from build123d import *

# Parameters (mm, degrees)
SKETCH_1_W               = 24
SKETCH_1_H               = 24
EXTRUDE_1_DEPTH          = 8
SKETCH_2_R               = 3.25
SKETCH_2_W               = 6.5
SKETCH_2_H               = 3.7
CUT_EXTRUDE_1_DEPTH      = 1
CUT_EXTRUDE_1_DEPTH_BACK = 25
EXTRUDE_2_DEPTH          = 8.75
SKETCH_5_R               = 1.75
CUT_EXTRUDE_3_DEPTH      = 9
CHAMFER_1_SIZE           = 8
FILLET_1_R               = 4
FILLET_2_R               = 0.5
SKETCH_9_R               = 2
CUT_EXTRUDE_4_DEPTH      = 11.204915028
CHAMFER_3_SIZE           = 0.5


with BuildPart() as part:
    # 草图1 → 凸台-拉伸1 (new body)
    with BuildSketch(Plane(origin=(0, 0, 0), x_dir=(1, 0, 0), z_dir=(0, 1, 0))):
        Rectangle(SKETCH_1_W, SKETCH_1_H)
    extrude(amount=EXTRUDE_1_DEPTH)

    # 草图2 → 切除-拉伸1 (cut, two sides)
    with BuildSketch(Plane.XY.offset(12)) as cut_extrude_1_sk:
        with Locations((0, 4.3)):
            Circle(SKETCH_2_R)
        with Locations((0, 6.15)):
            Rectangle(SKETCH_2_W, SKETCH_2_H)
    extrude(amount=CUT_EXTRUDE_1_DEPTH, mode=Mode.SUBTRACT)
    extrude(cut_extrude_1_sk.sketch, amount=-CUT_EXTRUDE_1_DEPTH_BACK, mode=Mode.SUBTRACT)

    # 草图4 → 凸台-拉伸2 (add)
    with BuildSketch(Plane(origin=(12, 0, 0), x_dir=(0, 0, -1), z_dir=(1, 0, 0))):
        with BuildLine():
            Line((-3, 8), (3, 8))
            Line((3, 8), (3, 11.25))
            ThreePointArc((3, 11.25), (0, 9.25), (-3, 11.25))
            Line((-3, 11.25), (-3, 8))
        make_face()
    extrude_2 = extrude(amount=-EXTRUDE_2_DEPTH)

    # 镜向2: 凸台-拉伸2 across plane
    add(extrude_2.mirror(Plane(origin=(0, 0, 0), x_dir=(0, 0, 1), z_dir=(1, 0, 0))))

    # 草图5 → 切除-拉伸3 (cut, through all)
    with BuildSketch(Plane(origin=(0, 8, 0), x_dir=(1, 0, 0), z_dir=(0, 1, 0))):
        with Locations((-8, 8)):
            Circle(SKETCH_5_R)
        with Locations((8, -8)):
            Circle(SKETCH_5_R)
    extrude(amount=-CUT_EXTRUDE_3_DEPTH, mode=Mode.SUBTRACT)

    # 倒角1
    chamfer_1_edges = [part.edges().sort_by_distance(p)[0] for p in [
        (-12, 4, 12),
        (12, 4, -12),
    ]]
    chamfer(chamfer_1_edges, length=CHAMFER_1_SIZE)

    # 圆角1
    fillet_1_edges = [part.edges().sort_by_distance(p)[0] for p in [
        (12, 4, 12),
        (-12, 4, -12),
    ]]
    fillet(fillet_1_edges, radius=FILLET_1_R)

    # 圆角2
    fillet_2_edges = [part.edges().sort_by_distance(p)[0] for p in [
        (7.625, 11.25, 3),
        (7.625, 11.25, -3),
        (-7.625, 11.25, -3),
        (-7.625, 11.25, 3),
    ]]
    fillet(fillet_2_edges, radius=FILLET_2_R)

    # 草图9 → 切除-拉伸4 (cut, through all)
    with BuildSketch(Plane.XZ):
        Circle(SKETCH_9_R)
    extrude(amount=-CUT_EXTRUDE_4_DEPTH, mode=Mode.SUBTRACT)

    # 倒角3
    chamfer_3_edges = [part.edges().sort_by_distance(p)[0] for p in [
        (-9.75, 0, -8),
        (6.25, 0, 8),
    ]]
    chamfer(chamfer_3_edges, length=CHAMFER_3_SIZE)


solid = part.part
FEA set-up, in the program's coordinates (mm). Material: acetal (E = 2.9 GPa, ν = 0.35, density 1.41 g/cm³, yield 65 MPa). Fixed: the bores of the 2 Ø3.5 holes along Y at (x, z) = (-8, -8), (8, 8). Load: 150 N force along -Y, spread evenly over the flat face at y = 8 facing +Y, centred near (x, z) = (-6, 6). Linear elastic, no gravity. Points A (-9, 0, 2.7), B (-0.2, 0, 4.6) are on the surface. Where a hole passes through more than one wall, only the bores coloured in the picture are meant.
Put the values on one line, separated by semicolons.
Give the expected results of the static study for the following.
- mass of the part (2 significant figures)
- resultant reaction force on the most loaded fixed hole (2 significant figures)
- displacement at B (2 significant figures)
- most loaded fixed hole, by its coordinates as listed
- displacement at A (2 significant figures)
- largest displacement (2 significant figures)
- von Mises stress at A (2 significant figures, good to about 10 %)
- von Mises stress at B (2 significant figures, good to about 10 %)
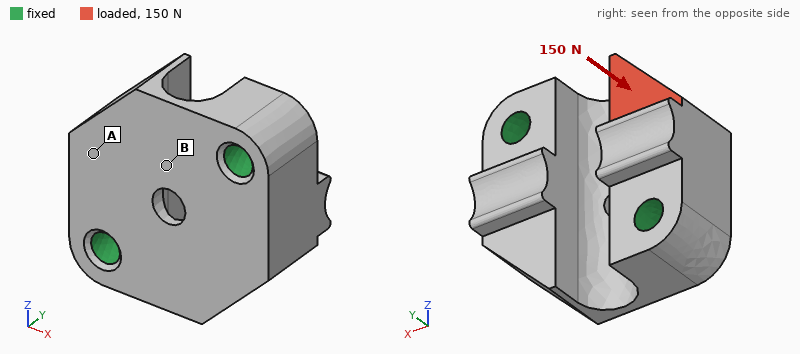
4.3 g; 120 N; 0.046 mm; (-8, -8); 0.076 mm; 0.16 mm; 3.4 MPa; 9.1 MPa
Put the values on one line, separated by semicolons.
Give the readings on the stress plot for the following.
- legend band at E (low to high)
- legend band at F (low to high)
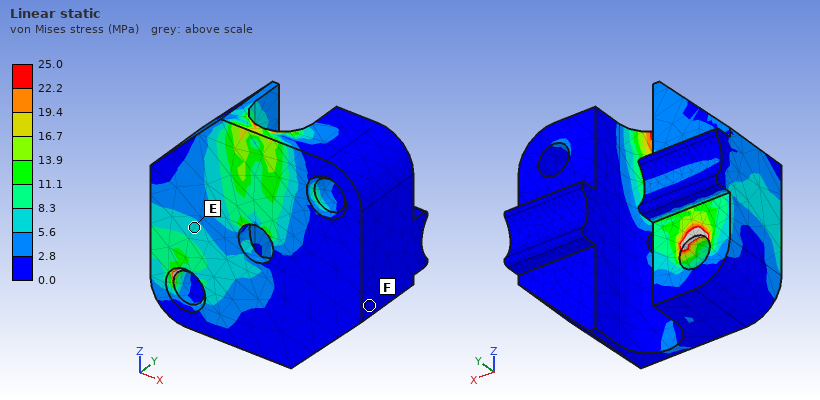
5.6 to 8.3 MPa; 0.0 to 2.8 MPa
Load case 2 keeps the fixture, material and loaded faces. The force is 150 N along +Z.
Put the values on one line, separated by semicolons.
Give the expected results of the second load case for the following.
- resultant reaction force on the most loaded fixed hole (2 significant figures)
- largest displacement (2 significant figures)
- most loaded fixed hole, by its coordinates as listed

150 N; 95 µm; (-8, -8)
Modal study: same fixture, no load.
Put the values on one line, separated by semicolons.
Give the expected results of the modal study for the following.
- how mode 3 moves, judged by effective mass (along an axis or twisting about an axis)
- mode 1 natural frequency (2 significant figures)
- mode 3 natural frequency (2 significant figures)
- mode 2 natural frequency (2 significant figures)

along X; 6600 Hz; 9000 Hz; 6800 Hz
